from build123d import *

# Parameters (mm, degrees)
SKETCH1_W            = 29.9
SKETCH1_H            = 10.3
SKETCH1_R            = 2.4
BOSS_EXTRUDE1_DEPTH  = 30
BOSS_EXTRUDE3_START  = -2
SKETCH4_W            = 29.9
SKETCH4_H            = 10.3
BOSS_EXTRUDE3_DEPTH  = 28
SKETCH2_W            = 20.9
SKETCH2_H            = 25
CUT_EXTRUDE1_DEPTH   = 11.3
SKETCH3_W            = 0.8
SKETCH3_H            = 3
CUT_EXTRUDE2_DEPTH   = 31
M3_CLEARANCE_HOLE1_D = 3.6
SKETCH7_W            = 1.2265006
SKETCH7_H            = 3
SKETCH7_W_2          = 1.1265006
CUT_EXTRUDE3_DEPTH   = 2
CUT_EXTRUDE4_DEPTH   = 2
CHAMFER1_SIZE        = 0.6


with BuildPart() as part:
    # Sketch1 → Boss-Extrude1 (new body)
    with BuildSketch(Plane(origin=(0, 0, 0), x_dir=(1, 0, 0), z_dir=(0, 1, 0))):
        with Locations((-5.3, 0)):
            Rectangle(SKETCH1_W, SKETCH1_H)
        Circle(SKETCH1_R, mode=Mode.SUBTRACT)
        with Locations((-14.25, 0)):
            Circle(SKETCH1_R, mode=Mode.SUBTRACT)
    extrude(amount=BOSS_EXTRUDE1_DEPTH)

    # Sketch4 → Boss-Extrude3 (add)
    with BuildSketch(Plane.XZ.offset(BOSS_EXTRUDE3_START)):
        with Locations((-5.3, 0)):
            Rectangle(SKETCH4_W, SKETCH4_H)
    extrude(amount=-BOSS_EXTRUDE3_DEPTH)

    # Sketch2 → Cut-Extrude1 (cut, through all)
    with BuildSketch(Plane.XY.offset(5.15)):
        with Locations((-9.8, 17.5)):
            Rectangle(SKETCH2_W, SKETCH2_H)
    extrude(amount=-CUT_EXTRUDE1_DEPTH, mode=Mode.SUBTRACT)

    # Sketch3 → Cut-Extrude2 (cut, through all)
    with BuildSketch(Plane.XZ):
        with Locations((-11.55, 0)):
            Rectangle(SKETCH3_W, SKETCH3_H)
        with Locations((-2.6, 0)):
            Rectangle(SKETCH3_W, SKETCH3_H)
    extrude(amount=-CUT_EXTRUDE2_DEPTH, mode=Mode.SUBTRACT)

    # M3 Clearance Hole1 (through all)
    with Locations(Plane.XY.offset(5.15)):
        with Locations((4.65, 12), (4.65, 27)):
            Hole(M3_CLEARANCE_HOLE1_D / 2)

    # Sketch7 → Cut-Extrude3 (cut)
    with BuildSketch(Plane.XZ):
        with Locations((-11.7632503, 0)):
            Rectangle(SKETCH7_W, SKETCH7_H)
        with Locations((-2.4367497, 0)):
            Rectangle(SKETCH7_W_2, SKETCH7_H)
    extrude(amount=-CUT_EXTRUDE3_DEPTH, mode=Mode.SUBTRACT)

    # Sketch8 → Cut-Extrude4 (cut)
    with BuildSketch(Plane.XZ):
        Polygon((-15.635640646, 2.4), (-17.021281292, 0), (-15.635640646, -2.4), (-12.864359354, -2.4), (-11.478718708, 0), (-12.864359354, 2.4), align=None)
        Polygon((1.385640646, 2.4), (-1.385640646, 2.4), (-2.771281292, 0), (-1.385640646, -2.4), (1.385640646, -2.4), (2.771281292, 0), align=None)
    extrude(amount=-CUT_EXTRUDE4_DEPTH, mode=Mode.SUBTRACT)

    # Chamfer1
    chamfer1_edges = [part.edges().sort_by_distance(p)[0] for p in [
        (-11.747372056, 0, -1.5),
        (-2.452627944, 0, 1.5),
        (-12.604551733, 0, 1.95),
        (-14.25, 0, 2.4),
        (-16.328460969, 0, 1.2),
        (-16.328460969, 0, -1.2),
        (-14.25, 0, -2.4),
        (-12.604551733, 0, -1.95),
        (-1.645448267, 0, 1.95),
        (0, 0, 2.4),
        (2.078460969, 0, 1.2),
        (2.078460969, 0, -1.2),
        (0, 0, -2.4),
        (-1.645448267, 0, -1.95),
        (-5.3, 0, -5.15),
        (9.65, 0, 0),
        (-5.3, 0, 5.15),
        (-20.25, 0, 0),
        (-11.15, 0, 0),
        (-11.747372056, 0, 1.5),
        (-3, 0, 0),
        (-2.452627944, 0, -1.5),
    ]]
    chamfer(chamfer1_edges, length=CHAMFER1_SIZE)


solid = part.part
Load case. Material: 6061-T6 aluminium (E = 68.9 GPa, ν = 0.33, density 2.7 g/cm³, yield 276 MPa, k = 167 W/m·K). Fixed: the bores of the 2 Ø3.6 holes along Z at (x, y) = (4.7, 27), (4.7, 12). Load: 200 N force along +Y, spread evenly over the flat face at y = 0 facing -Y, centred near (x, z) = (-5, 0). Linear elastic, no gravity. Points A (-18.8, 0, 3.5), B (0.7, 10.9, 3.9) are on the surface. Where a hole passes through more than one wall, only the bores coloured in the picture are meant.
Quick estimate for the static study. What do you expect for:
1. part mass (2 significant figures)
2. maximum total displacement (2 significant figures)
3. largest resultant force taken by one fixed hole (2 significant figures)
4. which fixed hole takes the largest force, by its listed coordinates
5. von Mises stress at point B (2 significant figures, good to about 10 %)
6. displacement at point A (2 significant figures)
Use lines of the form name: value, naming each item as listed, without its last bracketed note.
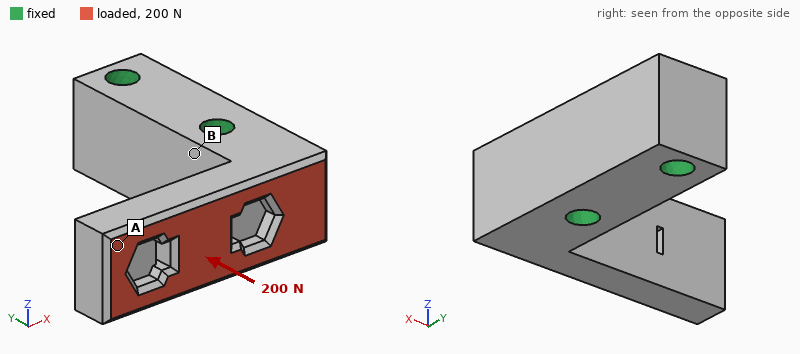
part mass: 9.5 g
maximum total displacement: 56 µm
largest resultant force taken by one fixed hole: 220 N
which fixed hole takes the largest force, by its listed coordinates: (4.7, 12)
von Mises stress at point B: 11 MPa
displacement at point A: 52 µm
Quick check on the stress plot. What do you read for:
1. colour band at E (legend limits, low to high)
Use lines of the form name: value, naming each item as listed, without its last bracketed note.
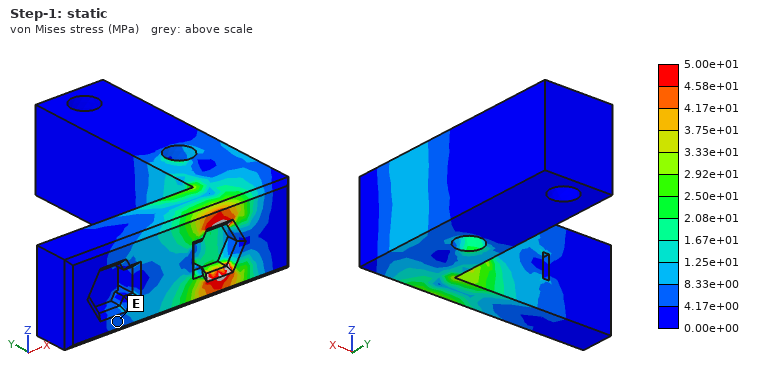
colour band at E: 4.17e+00 to 8.33e+00 MPa
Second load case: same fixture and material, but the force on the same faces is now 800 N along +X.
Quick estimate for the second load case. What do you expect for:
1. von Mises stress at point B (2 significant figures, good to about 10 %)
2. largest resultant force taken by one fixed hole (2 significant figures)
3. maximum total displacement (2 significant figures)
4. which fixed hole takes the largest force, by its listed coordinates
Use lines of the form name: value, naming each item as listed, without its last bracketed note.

von Mises stress at point B: 49 MPa
largest resultant force taken by one fixed hole: 1.0 kN
maximum total displacement: 0.10 mm
which fixed hole takes the largest force, by its listed coordinates: (4.7, 12)
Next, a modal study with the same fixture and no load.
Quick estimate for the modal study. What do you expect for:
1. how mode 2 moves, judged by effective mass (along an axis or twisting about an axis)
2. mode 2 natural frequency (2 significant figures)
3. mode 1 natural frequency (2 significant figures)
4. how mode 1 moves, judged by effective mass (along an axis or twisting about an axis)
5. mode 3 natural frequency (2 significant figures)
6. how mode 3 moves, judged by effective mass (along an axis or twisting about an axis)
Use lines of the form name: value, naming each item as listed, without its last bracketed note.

how mode 2 moves, judged by effective mass: along Z
mode 2 natural frequency: 8900 Hz
mode 1 natural frequency: 5800 Hz
how mode 1 moves, judged by effective mass: along Y
mode 3 natural frequency: 21 kHz
how mode 3 moves, judged by effective mass: along X
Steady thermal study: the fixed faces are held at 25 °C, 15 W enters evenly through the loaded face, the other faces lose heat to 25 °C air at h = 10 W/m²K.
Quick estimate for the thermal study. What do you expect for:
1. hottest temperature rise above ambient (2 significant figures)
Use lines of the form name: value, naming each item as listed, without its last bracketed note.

hottest temperature rise above ambient: 26 K
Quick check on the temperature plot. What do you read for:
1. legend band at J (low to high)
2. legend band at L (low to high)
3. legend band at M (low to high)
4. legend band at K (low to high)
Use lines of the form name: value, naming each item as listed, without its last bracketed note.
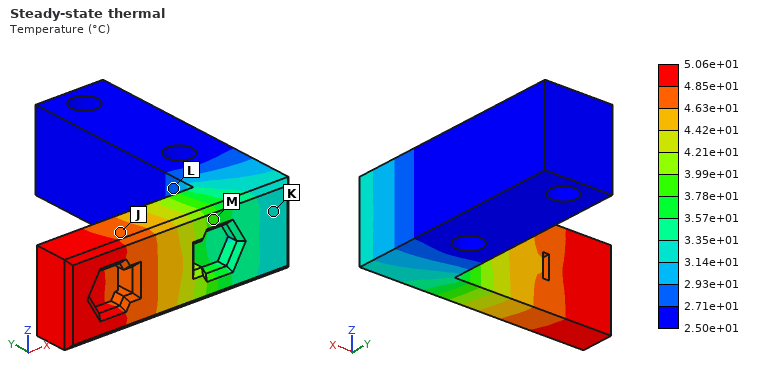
legend band at J: 4.63e+01 to 4.85e+01 °C
legend band at L: 2.71e+01 to 2.93e+01 °C
legend band at M: 3.78e+01 to 3.99e+01 °C
legend band at K: 3.14e+01 to 3.35e+01 °C
